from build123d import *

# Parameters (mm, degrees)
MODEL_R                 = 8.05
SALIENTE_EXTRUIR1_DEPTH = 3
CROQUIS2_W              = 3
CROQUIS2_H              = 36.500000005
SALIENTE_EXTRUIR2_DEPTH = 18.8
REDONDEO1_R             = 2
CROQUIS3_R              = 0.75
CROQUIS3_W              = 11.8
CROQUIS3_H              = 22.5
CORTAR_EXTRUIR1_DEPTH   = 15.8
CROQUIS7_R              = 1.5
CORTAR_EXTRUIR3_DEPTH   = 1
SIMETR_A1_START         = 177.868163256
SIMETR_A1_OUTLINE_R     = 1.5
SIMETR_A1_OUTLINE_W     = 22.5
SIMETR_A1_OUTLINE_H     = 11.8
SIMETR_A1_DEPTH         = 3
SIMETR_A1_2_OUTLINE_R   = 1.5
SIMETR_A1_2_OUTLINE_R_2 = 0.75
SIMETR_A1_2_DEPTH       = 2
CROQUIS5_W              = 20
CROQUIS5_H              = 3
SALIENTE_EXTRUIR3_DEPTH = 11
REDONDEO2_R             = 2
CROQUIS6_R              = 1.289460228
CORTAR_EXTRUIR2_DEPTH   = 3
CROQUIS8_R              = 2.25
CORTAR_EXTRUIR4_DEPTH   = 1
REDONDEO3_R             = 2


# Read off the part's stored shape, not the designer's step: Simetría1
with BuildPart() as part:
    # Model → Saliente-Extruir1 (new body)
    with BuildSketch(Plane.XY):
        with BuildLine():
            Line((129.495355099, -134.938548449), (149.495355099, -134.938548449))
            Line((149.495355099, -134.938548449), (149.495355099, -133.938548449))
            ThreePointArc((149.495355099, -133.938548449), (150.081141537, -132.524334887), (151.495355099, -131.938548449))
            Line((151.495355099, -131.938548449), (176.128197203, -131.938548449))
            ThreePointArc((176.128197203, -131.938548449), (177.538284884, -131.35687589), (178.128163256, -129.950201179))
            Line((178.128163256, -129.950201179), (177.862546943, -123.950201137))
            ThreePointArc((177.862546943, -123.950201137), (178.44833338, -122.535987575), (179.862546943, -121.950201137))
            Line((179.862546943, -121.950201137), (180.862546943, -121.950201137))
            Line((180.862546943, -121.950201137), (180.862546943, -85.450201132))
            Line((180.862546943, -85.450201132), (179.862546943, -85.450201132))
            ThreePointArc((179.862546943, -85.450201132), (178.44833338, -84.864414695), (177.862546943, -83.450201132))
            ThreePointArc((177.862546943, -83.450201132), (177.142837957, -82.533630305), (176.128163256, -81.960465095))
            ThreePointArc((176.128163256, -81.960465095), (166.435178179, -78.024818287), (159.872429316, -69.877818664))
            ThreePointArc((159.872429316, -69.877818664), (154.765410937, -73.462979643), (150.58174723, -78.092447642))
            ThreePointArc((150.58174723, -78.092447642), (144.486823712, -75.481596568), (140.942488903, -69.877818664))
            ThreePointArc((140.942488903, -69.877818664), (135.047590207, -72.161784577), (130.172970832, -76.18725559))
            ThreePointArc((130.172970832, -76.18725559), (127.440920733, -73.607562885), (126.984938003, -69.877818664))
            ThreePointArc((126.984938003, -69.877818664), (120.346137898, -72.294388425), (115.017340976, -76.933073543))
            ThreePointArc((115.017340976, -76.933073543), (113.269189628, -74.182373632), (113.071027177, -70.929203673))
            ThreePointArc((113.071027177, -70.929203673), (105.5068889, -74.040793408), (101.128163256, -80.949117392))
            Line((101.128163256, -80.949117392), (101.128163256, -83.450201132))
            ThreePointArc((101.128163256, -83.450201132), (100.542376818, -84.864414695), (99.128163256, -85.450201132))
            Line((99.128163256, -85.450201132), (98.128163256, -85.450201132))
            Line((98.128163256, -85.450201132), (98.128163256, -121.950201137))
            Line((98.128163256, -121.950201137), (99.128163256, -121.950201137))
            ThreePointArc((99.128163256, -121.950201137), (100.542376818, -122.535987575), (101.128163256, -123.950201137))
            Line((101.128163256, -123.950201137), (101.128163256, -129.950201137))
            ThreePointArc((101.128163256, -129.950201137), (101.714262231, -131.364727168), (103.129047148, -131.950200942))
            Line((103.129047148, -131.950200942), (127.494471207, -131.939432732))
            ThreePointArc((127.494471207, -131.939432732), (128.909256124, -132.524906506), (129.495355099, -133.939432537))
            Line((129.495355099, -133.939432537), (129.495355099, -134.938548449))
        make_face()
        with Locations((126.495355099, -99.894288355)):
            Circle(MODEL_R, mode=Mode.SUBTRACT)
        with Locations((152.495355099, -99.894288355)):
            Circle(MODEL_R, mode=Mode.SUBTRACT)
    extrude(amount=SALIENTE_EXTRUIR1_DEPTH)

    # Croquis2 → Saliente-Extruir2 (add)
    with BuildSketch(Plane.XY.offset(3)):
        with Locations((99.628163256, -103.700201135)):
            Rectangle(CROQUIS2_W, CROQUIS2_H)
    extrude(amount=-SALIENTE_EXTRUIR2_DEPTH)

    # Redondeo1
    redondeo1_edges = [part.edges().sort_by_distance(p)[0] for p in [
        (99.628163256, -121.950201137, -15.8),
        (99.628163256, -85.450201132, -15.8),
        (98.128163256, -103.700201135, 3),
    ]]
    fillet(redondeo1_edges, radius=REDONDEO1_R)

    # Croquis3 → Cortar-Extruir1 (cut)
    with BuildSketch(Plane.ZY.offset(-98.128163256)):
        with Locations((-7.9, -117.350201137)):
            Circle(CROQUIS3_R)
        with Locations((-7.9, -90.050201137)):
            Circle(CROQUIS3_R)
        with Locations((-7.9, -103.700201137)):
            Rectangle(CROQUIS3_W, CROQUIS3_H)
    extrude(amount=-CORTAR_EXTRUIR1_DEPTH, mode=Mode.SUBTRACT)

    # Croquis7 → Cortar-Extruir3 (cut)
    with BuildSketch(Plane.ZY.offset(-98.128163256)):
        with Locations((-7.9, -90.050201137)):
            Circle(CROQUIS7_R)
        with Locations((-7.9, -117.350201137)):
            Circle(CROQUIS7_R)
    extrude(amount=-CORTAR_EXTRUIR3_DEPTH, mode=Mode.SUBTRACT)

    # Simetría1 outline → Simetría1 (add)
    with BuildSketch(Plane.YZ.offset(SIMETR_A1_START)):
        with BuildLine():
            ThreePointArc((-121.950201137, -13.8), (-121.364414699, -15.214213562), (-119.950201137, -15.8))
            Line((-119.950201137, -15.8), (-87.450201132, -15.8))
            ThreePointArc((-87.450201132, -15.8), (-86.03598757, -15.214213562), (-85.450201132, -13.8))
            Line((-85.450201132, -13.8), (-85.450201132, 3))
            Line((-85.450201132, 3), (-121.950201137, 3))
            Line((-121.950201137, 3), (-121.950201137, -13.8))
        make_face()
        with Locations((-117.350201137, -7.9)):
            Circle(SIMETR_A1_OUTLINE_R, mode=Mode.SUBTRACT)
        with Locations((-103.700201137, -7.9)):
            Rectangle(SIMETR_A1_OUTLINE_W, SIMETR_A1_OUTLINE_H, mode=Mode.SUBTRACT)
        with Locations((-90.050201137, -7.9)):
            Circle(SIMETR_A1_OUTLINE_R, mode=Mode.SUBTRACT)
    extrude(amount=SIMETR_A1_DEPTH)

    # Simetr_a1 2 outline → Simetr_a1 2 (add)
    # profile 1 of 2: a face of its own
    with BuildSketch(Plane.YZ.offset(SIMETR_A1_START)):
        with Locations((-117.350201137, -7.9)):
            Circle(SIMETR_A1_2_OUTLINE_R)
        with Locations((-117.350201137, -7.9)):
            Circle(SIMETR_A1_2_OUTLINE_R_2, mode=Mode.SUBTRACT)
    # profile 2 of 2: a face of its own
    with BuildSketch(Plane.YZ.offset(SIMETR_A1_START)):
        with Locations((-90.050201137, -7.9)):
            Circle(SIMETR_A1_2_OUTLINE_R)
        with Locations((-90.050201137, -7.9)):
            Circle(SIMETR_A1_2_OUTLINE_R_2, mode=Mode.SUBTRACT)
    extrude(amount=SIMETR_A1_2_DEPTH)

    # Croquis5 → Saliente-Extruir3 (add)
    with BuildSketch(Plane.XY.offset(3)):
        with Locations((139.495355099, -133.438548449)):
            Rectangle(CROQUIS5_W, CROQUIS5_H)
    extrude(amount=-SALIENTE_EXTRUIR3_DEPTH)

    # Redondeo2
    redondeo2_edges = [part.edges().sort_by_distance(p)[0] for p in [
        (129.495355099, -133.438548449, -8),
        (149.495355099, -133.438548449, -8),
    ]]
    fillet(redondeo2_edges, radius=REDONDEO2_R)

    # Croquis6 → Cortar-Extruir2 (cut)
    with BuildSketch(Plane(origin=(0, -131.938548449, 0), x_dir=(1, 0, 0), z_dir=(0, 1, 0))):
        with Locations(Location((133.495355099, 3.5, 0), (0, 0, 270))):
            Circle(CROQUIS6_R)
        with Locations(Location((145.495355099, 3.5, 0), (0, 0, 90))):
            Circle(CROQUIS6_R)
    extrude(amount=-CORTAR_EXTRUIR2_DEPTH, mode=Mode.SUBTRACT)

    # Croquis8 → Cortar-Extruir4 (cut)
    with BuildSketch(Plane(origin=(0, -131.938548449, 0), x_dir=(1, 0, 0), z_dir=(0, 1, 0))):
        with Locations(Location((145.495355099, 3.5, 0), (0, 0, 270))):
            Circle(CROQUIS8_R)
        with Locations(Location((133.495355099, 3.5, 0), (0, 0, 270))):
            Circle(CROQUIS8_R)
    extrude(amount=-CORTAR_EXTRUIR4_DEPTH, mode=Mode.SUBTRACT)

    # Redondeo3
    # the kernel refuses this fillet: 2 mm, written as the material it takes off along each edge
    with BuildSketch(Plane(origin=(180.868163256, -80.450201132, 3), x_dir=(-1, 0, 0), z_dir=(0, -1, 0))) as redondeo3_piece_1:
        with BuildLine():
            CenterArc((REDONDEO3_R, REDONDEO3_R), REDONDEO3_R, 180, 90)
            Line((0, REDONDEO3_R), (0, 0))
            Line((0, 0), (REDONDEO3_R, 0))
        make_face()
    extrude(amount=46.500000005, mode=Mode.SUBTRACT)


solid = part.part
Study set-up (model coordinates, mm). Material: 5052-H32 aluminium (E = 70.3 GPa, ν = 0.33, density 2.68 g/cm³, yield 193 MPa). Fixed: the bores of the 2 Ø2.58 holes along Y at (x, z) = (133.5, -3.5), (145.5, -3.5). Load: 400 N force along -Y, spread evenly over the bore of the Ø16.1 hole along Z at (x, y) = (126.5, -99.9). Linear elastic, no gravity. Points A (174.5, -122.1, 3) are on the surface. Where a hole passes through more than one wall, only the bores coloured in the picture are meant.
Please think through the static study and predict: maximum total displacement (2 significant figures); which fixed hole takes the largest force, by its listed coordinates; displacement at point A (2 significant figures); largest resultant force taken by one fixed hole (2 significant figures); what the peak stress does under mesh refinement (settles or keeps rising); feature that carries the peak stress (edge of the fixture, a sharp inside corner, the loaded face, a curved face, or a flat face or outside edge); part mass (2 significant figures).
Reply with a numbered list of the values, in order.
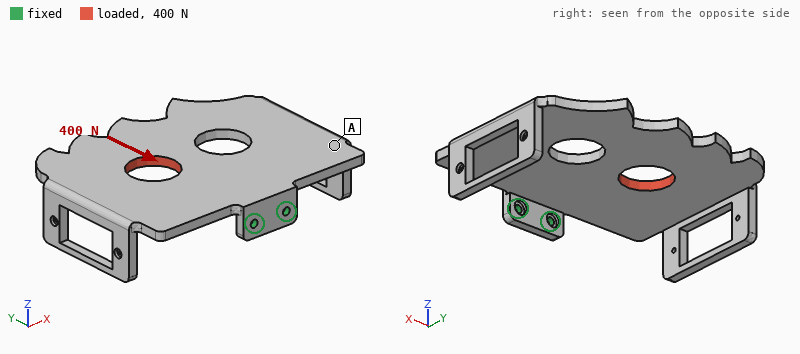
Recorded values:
1. 0.25 mm
2. (133.5, -3.5)
3. 0.053 mm
4. 580 N
5. keeps rising
6. edge of the fixture
7. 40 g
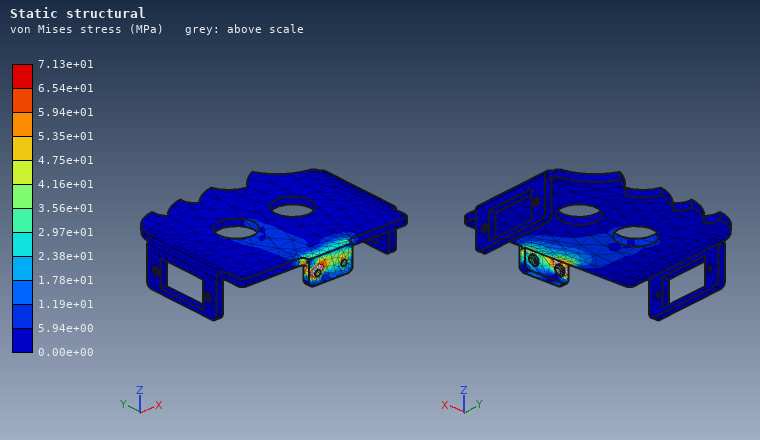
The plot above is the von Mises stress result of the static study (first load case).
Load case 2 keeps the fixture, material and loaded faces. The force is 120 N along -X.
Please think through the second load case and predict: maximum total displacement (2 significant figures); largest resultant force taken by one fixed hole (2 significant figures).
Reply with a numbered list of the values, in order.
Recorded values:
1. 0.11 mm
2. 310 N
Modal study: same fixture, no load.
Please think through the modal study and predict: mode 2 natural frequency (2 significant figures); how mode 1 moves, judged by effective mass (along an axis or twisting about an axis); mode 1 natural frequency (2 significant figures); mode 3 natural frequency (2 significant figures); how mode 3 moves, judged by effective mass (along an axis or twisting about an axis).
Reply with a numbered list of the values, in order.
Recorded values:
1. 590 Hz
2. along Z
3. 360 Hz
4. 1100 Hz
5. along X
